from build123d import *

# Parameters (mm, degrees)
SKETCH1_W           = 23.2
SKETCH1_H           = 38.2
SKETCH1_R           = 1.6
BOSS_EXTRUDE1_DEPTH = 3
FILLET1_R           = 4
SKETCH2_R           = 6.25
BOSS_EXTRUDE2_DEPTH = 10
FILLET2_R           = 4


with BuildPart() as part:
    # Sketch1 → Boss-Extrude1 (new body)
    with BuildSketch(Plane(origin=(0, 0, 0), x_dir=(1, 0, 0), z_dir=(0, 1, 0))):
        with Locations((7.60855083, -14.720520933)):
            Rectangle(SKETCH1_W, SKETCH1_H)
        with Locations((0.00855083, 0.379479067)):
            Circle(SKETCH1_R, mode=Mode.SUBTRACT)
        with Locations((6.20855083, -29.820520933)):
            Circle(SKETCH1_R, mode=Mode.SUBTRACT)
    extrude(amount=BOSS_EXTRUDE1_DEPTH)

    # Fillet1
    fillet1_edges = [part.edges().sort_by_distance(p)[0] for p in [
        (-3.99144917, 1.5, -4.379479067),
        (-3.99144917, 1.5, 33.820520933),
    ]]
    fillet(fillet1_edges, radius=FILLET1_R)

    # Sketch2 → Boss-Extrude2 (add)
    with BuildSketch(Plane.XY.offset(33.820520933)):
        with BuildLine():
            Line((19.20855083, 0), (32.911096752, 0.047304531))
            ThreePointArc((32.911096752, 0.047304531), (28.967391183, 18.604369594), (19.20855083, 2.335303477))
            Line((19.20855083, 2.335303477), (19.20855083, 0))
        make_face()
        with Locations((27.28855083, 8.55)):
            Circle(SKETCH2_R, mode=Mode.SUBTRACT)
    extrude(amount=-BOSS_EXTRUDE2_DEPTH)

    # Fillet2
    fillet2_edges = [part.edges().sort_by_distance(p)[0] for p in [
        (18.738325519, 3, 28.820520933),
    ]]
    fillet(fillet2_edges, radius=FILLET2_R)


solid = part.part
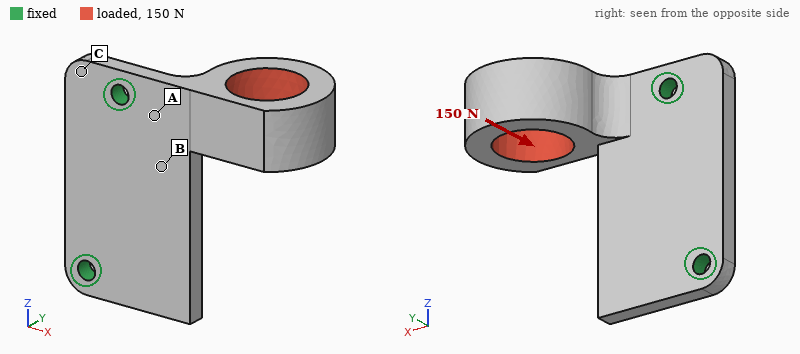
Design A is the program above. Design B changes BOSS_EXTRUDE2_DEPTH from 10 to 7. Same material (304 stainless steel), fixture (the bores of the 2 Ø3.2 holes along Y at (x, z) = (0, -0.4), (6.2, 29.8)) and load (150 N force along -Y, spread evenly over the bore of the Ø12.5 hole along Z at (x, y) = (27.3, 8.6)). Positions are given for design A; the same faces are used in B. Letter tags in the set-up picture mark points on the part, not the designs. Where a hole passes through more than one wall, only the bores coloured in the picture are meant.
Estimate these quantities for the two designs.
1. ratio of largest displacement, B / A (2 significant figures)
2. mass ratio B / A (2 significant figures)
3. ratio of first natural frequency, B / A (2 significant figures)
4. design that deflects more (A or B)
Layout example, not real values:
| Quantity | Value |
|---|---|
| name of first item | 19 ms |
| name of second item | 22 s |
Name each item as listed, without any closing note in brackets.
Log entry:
| Quantity | Value |
|---|---|
| ratio of largest displacement, B / A | 1.2 |
| mass ratio B / A | 0.87 |
| ratio of first natural frequency, B / A | 1.1 |
| design that deflects more | B |
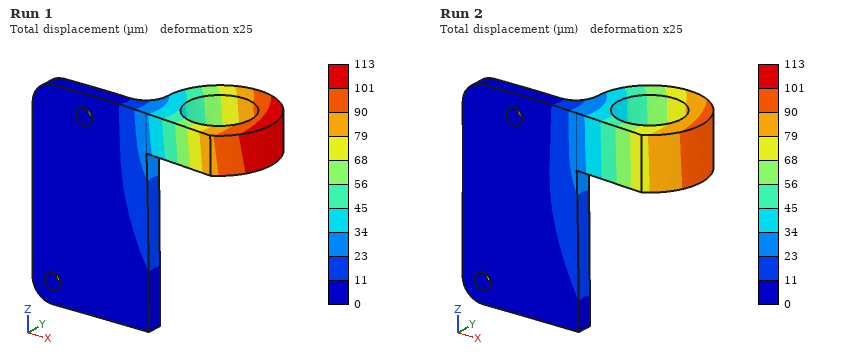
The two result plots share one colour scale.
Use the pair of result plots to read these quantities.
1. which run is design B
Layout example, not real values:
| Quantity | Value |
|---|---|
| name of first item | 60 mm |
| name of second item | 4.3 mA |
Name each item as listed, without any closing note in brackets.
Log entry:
| Quantity | Value |
|---|---|
| which run is design B | Run 1 |
